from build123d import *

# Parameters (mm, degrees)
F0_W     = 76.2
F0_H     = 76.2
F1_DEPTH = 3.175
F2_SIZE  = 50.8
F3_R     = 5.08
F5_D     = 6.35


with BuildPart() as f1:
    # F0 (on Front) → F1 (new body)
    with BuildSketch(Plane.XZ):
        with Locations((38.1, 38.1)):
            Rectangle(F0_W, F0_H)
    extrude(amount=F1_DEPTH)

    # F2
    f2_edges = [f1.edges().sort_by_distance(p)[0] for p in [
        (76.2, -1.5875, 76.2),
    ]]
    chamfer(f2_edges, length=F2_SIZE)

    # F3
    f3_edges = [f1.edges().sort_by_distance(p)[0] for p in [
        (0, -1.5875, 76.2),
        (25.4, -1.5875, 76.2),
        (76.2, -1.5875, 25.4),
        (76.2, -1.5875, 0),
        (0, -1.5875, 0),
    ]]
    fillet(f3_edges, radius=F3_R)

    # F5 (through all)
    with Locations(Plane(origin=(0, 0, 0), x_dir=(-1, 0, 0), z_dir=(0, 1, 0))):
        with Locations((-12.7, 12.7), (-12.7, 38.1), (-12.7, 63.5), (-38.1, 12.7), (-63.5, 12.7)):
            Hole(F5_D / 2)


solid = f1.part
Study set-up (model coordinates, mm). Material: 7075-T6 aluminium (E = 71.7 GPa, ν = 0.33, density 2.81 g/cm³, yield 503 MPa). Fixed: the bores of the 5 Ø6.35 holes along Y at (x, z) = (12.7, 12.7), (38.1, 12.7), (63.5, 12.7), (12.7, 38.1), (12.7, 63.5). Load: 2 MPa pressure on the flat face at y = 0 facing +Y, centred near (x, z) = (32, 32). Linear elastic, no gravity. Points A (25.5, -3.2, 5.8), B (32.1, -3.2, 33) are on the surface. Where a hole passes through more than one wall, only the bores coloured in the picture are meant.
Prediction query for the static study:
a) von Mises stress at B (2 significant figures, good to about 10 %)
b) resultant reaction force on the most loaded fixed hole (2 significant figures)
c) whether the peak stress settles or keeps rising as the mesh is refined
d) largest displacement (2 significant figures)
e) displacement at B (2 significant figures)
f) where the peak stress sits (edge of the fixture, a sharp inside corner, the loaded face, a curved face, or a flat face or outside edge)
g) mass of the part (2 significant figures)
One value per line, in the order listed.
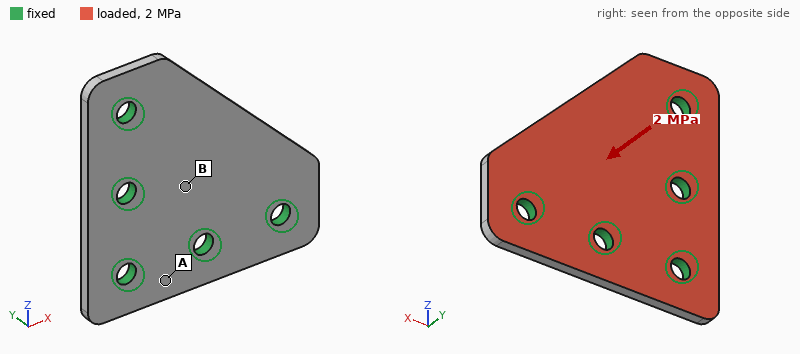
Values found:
120 MPa
2.0 kN
keeps rising
0.70 mm
0.16 mm
edge of the fixture
39 g
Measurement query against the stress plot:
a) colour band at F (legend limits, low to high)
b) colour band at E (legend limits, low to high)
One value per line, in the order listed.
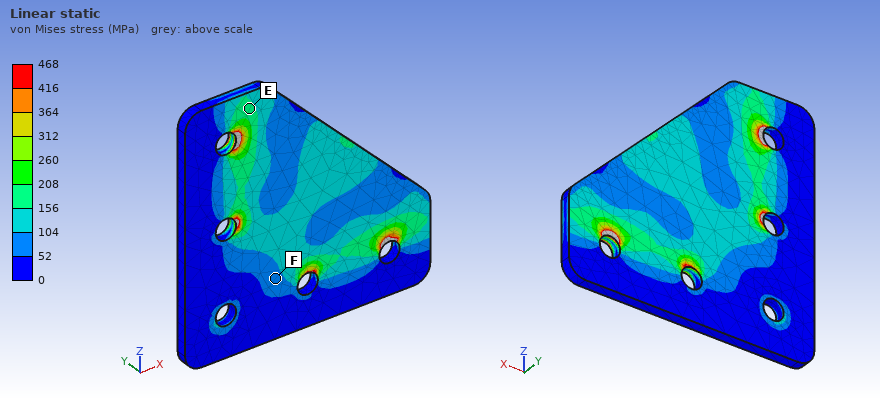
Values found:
52 to 104 MPa
156 to 208 MPa
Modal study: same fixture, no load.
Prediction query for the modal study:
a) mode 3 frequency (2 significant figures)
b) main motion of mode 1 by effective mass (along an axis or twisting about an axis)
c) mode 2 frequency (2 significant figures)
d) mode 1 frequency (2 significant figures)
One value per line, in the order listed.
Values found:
11 kHz
along Y
8200 Hz
3900 Hz
